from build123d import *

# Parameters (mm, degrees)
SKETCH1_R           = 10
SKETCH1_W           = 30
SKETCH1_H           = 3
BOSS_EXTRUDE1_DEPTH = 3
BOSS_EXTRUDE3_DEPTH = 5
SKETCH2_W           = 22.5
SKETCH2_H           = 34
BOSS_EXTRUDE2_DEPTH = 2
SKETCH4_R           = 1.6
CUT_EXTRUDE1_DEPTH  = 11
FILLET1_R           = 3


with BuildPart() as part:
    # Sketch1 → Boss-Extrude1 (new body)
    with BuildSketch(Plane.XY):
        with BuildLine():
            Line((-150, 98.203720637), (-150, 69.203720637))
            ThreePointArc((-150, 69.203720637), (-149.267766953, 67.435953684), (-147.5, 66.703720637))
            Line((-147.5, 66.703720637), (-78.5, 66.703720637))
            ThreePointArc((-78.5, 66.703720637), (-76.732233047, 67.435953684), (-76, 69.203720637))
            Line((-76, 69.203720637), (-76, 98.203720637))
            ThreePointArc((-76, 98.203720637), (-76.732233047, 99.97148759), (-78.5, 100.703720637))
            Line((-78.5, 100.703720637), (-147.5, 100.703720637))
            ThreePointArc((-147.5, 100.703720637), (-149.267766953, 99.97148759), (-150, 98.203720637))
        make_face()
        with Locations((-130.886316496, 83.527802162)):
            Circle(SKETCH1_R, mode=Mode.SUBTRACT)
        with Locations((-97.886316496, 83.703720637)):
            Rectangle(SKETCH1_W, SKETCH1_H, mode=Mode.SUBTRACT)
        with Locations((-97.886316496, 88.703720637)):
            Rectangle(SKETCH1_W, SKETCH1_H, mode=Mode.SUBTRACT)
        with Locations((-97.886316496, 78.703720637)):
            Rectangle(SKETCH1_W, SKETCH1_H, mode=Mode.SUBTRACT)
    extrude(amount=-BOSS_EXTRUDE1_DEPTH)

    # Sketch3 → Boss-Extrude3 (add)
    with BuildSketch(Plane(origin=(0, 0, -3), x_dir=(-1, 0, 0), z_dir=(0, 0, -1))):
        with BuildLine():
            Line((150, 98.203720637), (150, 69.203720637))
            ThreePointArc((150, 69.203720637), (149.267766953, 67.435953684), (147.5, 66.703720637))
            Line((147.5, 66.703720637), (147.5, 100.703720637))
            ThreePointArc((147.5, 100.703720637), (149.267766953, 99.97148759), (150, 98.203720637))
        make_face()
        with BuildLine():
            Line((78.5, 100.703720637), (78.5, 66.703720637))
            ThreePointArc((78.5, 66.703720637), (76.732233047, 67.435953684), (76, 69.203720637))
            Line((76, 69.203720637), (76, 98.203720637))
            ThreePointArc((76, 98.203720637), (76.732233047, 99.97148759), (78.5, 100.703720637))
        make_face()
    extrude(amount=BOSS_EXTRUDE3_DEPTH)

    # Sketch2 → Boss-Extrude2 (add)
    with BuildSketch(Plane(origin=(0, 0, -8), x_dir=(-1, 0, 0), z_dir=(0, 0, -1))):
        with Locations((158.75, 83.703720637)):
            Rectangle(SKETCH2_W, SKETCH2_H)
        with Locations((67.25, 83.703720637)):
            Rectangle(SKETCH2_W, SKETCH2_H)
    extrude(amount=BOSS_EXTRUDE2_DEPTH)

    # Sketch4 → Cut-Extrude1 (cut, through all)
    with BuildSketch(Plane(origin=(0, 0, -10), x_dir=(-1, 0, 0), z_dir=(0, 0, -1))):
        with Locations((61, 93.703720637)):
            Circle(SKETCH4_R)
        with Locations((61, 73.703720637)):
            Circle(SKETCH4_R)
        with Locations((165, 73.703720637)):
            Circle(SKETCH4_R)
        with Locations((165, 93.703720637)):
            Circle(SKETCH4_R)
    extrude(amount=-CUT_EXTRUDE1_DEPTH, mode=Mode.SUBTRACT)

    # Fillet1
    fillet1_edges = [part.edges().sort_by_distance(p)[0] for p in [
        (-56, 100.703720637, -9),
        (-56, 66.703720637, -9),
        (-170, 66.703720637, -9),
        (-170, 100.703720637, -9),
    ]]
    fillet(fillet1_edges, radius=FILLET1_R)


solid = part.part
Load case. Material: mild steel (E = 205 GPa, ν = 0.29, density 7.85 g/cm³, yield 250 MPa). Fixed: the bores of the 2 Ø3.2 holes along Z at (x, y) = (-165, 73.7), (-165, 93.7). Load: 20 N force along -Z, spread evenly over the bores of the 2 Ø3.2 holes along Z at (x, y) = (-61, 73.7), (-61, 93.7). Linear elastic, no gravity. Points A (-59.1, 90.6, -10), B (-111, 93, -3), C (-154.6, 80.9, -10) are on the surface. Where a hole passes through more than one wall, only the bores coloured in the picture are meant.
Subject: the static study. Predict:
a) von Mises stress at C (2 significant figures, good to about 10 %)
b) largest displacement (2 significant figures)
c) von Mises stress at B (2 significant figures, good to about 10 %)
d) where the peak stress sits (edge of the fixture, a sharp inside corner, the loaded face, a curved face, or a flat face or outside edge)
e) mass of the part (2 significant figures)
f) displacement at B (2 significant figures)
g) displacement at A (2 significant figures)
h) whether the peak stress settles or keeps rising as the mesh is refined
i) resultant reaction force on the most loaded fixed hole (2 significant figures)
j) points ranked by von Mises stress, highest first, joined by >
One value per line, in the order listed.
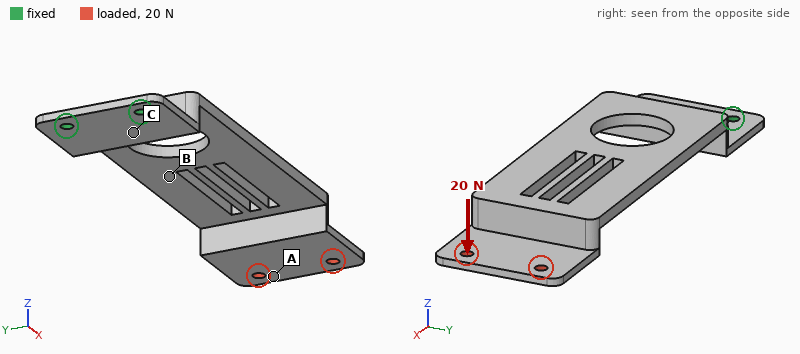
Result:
75 MPa
1.3 mm
26 MPa
edge of the fixture
75 g
0.45 mm
1.2 mm
keeps rising
15 N
C > B > A
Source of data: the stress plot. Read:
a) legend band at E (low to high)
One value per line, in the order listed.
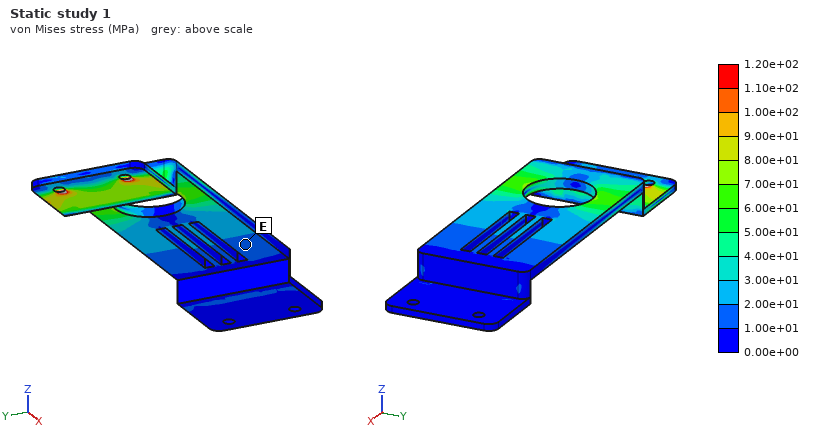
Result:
1.00e+01 to 2.00e+01 MPa
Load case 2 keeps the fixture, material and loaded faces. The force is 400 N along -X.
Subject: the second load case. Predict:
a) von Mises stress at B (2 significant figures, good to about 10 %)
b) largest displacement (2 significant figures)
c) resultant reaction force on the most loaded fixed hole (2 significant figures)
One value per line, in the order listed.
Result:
83 MPa
1.4 mm
200 N
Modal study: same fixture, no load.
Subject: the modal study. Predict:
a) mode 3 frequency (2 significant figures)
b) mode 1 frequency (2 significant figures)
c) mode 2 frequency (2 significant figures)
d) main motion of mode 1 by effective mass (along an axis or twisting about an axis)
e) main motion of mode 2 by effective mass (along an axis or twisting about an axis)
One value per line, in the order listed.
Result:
1000 Hz
140 Hz
700 Hz
along Z
along Y
